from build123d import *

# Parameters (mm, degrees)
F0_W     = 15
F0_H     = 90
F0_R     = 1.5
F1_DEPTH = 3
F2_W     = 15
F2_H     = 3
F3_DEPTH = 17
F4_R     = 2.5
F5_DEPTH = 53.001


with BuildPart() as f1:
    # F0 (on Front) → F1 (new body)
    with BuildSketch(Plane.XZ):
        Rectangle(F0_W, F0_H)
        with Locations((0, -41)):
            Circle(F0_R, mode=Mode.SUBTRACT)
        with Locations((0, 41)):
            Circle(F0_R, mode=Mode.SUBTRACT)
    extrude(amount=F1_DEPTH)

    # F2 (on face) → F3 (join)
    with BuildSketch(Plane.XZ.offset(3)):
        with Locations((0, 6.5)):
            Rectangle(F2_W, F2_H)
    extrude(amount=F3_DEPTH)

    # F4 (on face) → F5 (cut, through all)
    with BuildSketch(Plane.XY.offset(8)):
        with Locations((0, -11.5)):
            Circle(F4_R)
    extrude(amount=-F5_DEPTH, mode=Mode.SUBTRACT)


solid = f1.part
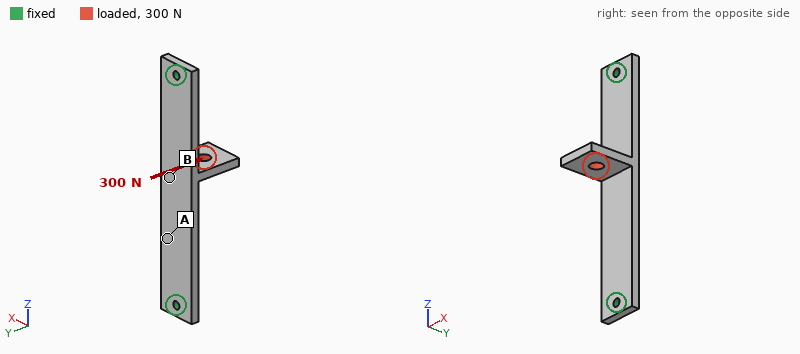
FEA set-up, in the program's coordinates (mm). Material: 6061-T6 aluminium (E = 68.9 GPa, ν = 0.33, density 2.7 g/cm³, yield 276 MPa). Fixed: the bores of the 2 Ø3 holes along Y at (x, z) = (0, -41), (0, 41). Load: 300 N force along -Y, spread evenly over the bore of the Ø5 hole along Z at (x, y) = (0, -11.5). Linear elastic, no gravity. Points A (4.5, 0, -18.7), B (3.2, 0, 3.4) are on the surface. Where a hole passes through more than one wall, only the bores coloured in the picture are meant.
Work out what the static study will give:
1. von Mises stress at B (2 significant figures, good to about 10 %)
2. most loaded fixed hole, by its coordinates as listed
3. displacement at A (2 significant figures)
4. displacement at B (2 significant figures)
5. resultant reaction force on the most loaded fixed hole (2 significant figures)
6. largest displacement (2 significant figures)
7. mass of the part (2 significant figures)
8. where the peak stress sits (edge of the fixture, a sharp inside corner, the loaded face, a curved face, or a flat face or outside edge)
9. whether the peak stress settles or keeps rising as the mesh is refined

110 MPa
(0, 41)
0.18 mm
0.34 mm
190 N
0.34 mm
13 g
edge of the fixture
keeps rising
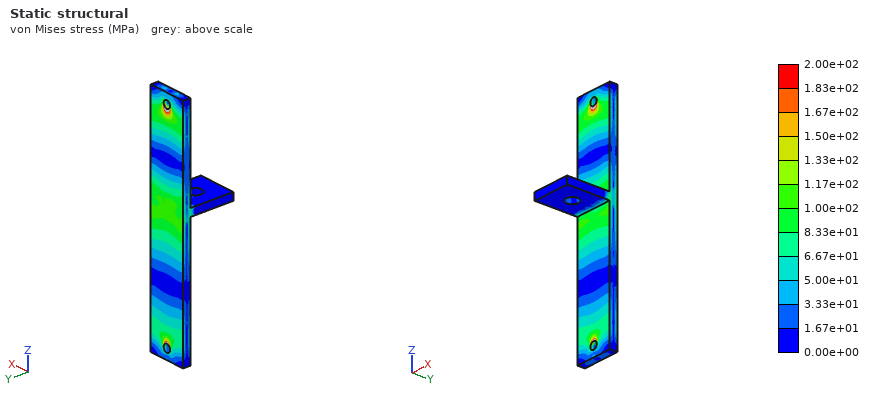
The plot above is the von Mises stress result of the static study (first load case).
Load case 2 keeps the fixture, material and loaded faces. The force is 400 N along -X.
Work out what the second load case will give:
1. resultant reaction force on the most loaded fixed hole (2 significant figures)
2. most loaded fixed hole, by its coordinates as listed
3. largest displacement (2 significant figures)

240 N
(0, 41)
0.52 mm
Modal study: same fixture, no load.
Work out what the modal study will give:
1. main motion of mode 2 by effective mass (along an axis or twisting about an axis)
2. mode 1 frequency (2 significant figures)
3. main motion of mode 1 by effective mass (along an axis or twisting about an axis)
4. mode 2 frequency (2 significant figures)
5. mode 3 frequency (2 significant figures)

along X
1900 Hz
along Y
3300 Hz
4600 Hz
